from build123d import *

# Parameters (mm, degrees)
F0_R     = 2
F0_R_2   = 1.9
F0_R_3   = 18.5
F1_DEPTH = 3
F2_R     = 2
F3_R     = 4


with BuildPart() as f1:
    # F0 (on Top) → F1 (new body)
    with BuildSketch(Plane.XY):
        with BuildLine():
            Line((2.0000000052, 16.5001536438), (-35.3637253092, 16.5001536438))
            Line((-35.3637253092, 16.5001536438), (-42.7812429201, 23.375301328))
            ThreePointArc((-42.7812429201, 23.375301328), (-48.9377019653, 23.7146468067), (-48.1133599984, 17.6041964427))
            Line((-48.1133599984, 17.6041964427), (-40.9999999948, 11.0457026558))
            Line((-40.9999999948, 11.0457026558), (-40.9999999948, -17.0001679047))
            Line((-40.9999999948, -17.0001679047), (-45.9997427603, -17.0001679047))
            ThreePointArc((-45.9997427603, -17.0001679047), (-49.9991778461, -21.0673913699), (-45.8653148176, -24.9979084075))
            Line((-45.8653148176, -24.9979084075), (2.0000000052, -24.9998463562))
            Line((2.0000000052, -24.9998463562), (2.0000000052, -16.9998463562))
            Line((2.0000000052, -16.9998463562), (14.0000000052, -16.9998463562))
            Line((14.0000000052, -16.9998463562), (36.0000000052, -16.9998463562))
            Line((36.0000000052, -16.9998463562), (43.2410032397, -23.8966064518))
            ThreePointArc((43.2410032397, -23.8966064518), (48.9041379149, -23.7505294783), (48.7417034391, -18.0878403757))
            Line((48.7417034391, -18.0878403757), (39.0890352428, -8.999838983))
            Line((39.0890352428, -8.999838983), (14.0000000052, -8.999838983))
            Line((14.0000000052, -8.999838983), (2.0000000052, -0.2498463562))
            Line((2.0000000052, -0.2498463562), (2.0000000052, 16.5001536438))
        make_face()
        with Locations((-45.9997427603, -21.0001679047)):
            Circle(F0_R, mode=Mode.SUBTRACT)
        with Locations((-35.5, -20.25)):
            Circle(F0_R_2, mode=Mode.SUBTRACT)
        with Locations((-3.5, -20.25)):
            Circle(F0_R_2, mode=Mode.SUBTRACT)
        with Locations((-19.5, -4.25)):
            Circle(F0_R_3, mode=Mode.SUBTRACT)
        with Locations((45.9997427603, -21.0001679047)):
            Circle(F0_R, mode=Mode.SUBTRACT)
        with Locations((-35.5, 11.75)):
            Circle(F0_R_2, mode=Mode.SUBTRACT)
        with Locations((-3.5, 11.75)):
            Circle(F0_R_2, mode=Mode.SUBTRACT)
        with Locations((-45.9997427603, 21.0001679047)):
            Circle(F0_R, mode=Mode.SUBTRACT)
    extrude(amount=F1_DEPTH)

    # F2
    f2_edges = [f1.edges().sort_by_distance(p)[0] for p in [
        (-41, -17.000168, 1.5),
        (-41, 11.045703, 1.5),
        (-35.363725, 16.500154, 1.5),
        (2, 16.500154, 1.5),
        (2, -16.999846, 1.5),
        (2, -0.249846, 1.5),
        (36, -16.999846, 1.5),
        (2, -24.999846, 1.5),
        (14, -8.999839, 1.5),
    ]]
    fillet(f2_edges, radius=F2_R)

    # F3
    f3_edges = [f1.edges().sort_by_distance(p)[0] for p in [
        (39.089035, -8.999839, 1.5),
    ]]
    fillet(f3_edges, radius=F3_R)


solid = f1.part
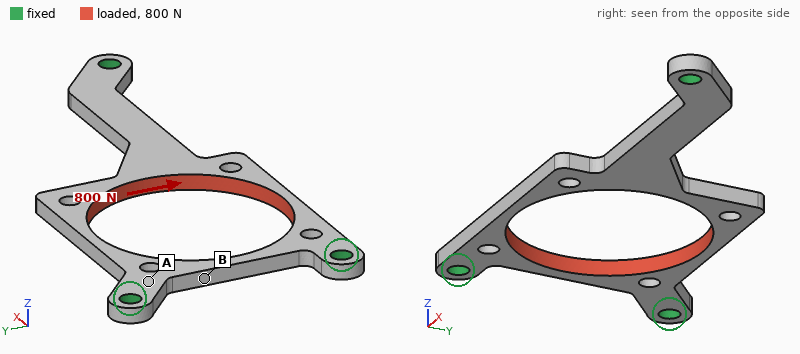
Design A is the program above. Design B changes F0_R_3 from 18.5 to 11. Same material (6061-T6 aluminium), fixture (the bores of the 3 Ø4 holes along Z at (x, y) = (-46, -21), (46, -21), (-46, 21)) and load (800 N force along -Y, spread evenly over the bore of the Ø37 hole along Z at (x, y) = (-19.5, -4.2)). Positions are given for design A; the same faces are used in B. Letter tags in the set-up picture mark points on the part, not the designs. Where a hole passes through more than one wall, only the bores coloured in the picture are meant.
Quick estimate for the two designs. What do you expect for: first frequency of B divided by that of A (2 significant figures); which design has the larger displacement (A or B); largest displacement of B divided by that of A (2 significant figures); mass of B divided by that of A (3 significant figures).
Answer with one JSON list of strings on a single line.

["0.95", "A", "0.13", "1.56"]
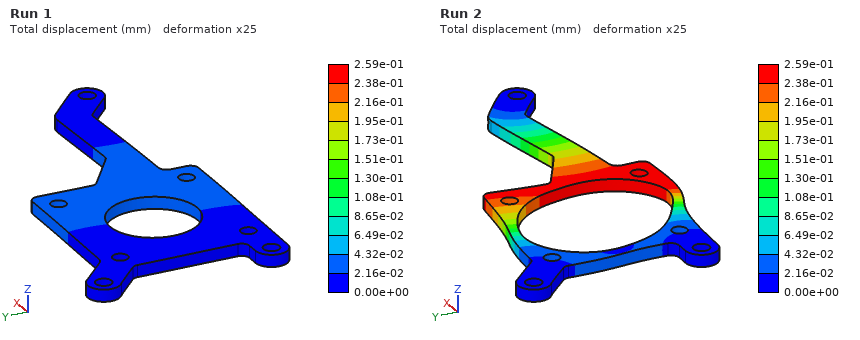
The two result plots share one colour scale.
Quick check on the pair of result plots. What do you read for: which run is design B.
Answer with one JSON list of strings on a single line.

["Run 1"]
